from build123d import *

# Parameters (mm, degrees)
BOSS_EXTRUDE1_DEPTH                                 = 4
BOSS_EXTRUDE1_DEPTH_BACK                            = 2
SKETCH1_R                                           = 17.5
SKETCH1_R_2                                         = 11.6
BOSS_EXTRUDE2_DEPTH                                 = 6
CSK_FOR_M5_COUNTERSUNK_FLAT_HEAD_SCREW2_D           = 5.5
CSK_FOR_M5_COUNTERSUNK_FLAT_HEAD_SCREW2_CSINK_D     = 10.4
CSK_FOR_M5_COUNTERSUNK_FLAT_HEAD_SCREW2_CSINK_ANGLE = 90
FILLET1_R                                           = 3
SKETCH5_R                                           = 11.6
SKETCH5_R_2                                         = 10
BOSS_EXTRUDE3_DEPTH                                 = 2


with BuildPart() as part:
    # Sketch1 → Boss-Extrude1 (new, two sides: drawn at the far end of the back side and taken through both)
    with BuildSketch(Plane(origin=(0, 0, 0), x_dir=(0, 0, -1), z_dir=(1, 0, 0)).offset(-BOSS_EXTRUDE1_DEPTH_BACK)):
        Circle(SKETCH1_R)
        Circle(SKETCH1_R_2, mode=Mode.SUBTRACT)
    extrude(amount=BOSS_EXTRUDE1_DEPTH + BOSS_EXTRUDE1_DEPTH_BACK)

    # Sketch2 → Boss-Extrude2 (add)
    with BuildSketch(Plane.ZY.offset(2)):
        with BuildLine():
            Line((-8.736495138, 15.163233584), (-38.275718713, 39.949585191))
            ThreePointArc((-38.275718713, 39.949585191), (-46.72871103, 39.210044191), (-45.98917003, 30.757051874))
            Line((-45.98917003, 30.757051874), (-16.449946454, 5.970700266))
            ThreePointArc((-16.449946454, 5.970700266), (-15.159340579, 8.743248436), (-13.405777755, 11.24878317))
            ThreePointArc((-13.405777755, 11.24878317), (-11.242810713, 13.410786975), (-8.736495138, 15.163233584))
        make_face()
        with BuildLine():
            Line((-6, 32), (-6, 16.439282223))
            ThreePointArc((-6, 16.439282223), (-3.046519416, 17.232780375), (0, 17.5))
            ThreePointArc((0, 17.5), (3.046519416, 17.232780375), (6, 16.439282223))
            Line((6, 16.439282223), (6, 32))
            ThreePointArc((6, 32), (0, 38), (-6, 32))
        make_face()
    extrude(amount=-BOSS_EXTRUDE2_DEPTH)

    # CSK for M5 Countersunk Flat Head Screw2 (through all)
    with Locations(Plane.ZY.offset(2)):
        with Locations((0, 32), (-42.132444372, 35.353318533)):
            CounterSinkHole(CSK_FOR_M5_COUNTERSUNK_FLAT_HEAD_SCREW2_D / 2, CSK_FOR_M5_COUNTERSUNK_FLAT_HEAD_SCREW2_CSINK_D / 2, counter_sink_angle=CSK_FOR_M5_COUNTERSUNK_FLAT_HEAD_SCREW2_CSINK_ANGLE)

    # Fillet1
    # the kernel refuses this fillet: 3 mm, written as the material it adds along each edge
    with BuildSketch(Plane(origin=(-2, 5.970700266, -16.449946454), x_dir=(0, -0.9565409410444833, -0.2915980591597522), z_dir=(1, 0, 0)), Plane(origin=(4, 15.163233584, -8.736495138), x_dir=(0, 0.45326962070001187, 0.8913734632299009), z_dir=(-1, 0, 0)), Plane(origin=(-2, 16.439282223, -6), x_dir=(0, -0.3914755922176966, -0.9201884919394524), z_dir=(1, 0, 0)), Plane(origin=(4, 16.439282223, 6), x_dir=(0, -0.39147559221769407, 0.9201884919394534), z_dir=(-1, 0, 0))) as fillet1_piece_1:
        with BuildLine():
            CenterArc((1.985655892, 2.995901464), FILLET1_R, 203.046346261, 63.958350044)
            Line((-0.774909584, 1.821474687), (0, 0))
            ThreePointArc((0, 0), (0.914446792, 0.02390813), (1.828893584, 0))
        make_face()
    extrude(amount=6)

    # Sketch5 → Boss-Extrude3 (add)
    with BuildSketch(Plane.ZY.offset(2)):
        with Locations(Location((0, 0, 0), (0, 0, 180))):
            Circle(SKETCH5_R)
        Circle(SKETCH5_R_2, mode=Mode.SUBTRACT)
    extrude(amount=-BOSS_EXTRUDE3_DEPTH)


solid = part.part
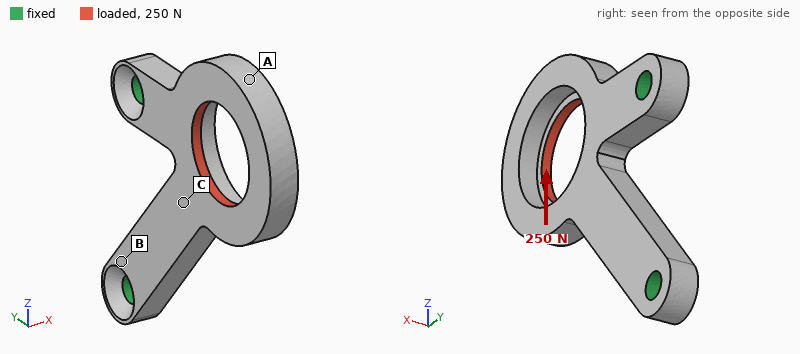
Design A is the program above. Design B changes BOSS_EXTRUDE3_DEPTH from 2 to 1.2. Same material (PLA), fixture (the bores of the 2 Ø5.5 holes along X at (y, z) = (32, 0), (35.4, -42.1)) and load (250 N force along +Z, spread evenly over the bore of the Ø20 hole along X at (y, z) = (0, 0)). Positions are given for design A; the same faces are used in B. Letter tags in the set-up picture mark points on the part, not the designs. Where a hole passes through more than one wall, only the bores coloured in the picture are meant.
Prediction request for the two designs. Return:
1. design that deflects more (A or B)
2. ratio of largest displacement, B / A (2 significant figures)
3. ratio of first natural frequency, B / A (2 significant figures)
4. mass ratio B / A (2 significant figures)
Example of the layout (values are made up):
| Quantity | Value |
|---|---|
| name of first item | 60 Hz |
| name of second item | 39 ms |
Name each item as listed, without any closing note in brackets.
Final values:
| Quantity | Value |
|---|---|
| design that deflects more | B |
| ratio of largest displacement, B / A | 1.1 |
| ratio of first natural frequency, B / A | 1.0 |
| mass ratio B / A | 0.99 |
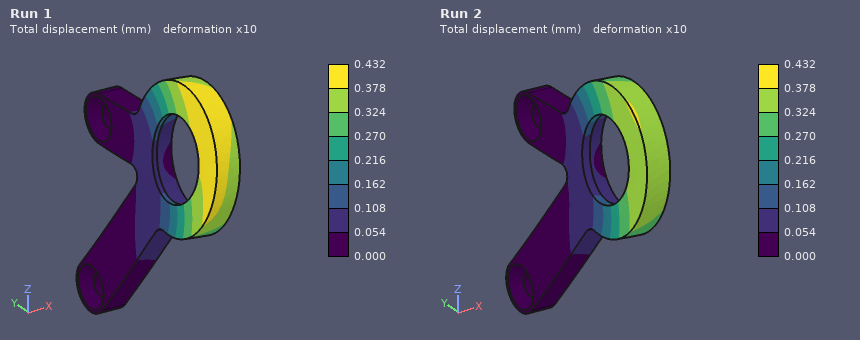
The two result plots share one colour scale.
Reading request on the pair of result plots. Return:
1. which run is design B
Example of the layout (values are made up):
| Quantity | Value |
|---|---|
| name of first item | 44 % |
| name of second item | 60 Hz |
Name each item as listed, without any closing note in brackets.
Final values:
| Quantity | Value |
|---|---|
| which run is design B | Run 1 |
